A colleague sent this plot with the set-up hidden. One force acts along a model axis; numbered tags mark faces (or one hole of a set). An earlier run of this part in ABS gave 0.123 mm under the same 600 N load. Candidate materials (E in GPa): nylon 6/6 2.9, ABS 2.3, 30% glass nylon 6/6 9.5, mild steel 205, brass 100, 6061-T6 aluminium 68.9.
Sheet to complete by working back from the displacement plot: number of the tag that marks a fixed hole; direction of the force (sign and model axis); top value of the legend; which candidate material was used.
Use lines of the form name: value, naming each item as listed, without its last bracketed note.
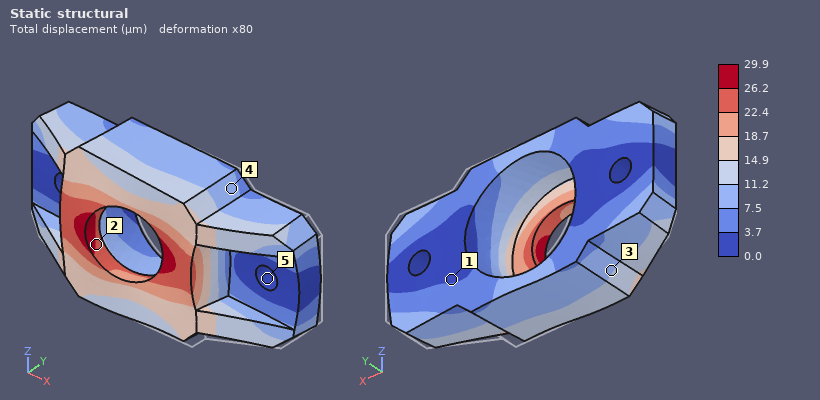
number of the tag that marks a fixed hole: 5
direction of the force: -X
top value of the legend: 29.9 µm
which candidate material was used: 30% glass nylon 6/6
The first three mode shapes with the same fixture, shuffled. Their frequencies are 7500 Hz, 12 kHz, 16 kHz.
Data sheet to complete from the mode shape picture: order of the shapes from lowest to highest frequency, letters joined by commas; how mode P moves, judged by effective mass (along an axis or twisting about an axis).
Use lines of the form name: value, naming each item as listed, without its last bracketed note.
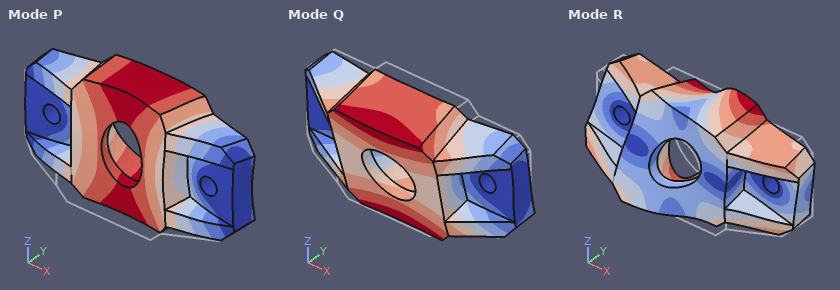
order of the shapes from lowest to highest frequency, letters joined by commas: Q, P, R
how mode P moves, judged by effective mass: along Y
